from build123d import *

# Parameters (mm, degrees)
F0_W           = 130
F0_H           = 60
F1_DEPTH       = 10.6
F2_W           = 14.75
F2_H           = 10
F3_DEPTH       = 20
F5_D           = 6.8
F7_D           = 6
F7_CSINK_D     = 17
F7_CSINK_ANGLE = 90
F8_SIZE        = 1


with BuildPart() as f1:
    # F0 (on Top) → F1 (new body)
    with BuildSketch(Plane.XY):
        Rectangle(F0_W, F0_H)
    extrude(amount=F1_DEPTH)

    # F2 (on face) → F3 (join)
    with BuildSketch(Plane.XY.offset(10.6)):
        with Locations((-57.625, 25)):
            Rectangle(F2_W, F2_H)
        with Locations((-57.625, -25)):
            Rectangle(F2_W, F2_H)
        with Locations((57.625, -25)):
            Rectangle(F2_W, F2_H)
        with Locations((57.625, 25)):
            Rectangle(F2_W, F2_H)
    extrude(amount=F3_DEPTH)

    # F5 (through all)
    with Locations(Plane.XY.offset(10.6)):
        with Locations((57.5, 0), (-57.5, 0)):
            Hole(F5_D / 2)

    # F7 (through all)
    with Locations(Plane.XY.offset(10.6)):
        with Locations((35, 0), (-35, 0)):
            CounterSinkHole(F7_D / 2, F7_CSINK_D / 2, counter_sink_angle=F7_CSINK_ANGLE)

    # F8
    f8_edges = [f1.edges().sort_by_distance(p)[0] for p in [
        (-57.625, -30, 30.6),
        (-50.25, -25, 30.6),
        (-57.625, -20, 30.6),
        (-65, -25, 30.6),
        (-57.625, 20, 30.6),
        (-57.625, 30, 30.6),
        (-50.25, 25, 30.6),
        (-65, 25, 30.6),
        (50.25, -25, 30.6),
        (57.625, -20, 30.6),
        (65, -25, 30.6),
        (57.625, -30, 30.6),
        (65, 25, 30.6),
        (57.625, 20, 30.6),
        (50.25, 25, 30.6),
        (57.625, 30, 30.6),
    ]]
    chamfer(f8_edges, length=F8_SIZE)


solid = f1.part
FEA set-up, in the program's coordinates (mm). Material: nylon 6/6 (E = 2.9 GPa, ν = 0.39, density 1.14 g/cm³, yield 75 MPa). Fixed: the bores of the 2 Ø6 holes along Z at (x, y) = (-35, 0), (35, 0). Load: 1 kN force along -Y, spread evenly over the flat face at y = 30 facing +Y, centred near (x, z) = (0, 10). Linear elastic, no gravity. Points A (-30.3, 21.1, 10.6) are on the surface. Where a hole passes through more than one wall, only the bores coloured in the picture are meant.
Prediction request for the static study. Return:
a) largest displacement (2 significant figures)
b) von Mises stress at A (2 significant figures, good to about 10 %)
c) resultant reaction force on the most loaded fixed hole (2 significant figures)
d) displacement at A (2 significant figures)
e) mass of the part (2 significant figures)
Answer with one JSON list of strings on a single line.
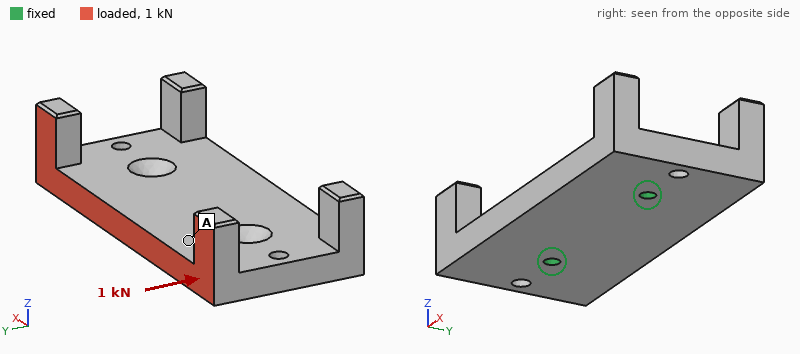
["0.55 mm", "1.9 MPa", "500 N", "0.18 mm", "100 g"]
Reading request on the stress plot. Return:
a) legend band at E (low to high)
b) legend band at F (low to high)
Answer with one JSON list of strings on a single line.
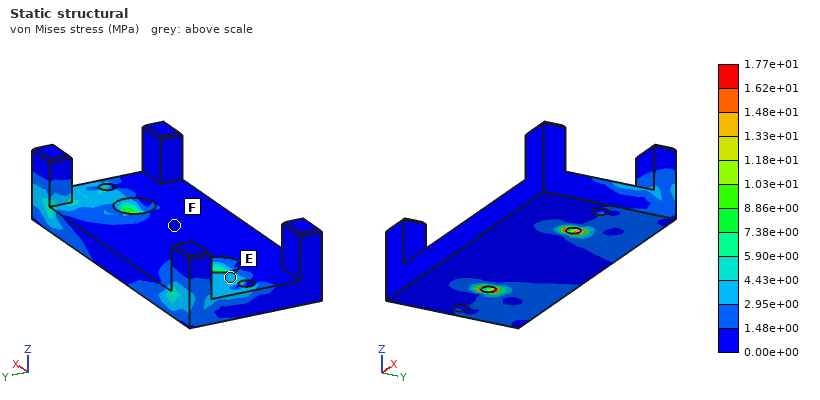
["2.95e+00 to 4.43e+00 MPa", "0.00e+00 to 1.48e+00 MPa"]
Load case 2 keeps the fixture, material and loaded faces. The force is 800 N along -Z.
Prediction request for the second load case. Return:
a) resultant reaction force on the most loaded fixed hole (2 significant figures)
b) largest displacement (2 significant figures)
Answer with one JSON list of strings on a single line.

["410 N", "1.5 mm"]
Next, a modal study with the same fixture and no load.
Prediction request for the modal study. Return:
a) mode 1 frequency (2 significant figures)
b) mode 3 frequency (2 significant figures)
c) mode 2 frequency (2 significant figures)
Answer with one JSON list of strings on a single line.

["720 Hz", "1100 Hz", "1000 Hz"]
